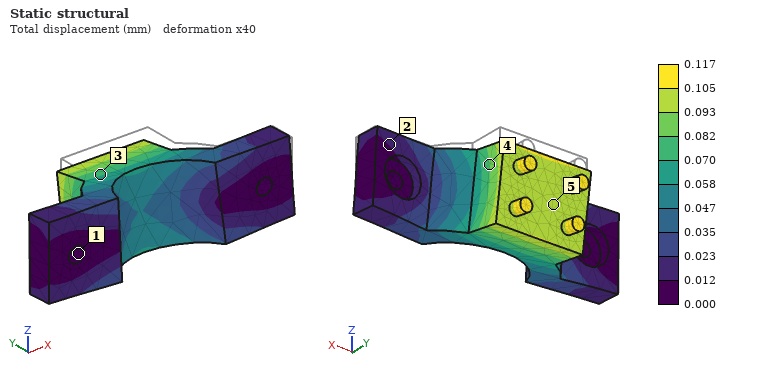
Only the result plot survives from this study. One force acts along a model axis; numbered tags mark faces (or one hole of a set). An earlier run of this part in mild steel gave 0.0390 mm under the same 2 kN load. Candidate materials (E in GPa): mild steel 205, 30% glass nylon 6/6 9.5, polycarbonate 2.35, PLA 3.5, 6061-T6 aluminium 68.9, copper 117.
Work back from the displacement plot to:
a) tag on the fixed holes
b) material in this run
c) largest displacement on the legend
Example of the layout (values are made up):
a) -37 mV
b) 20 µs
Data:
a) 1
b) 6061-T6 aluminium
c) 0.117 mm
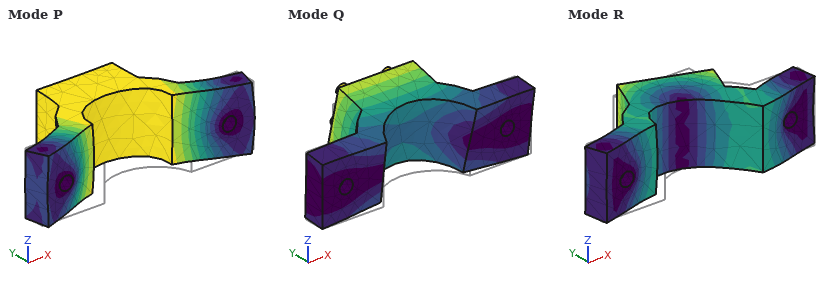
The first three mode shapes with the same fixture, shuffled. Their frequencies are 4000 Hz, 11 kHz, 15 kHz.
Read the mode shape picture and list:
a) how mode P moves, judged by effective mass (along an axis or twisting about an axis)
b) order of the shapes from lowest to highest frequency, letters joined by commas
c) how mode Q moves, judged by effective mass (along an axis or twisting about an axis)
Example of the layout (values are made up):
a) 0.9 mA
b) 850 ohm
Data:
a) along Y
b) Q, P, R
c) along Z
